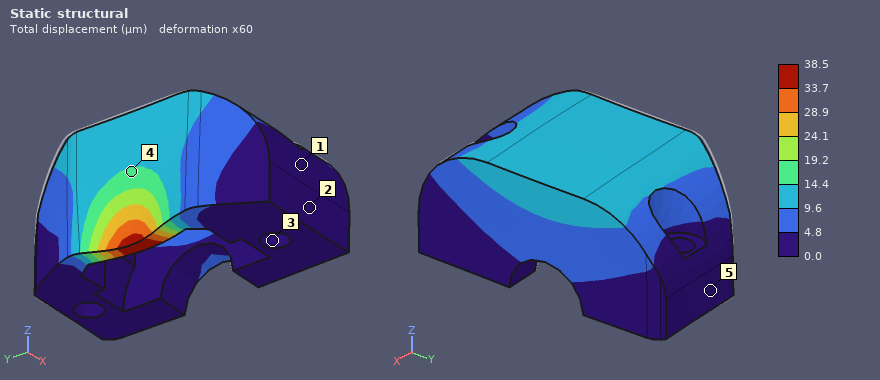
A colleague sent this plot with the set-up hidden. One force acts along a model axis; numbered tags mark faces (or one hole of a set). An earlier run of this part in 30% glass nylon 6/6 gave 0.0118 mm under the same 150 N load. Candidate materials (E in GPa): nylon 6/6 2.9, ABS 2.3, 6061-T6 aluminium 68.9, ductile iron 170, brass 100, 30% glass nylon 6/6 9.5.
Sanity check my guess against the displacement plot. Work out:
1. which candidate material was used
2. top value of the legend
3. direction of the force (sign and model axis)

nylon 6/6
38.5 µm
+X
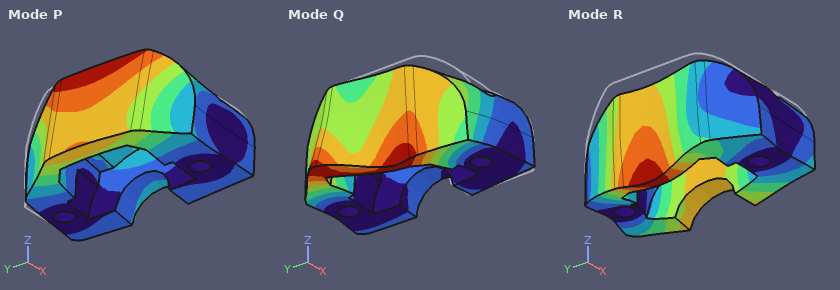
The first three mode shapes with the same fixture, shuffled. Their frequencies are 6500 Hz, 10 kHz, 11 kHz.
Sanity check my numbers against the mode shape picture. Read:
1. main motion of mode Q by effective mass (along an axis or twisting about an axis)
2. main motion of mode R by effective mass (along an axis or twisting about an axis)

along Y
along Z
